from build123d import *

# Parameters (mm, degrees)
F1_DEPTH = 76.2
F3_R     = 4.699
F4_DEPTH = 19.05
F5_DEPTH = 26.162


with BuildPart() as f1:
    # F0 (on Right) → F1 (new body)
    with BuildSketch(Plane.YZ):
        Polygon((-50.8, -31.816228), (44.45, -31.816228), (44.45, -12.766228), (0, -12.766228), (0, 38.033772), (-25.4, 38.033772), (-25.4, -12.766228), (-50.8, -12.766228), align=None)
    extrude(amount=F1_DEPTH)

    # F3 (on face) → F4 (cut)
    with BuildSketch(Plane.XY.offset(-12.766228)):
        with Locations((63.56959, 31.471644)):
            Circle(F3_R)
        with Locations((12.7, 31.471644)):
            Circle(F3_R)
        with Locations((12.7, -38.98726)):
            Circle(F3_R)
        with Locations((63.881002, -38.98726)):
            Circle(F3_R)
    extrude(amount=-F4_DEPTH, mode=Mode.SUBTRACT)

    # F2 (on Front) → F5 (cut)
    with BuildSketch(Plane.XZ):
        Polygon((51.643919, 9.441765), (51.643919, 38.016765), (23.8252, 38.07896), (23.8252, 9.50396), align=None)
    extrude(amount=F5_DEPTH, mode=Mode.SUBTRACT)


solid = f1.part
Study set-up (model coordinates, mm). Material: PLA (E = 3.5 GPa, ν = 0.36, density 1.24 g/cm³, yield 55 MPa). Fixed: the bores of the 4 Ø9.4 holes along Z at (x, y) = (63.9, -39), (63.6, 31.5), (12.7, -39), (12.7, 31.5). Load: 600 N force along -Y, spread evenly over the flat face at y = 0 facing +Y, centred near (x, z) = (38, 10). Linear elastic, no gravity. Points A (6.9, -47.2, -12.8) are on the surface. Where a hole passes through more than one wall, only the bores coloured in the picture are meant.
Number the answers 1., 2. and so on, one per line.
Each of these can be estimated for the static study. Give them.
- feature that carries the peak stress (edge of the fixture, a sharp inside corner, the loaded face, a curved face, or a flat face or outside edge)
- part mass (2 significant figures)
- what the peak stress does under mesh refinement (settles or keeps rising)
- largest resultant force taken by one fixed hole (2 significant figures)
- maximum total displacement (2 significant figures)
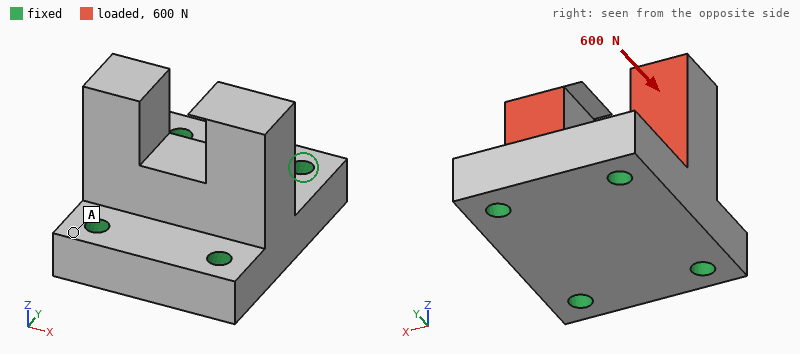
1. edge of the fixture
2. 260 g
3. keeps rising
4. 240 N
5. 72 µm
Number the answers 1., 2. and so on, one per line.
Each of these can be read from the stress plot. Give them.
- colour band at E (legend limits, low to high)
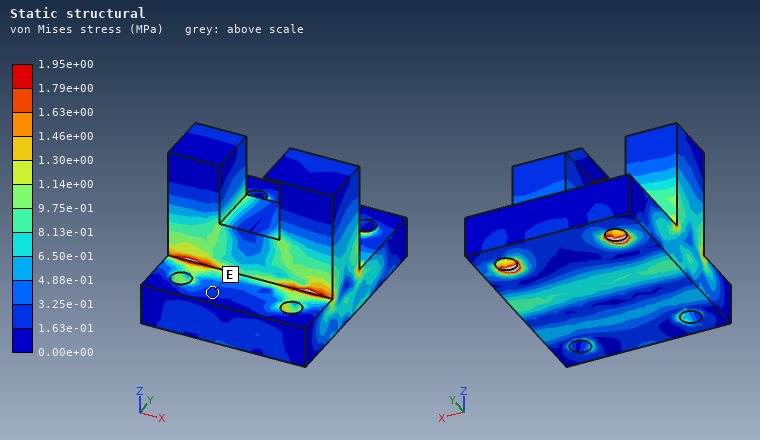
1. 1.63e-01 to 3.25e-01 MPa
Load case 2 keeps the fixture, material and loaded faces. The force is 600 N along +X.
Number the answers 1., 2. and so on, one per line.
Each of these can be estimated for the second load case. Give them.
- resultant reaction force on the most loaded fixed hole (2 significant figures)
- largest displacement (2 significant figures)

1. 340 N
2. 65 µm
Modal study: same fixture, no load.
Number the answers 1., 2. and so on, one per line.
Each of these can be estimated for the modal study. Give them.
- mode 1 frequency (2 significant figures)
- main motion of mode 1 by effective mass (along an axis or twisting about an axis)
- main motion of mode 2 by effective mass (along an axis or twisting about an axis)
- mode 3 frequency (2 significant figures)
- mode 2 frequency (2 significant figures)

1. 1800 Hz
2. along Y
3. along X
4. 2200 Hz
5. 2000 Hz
